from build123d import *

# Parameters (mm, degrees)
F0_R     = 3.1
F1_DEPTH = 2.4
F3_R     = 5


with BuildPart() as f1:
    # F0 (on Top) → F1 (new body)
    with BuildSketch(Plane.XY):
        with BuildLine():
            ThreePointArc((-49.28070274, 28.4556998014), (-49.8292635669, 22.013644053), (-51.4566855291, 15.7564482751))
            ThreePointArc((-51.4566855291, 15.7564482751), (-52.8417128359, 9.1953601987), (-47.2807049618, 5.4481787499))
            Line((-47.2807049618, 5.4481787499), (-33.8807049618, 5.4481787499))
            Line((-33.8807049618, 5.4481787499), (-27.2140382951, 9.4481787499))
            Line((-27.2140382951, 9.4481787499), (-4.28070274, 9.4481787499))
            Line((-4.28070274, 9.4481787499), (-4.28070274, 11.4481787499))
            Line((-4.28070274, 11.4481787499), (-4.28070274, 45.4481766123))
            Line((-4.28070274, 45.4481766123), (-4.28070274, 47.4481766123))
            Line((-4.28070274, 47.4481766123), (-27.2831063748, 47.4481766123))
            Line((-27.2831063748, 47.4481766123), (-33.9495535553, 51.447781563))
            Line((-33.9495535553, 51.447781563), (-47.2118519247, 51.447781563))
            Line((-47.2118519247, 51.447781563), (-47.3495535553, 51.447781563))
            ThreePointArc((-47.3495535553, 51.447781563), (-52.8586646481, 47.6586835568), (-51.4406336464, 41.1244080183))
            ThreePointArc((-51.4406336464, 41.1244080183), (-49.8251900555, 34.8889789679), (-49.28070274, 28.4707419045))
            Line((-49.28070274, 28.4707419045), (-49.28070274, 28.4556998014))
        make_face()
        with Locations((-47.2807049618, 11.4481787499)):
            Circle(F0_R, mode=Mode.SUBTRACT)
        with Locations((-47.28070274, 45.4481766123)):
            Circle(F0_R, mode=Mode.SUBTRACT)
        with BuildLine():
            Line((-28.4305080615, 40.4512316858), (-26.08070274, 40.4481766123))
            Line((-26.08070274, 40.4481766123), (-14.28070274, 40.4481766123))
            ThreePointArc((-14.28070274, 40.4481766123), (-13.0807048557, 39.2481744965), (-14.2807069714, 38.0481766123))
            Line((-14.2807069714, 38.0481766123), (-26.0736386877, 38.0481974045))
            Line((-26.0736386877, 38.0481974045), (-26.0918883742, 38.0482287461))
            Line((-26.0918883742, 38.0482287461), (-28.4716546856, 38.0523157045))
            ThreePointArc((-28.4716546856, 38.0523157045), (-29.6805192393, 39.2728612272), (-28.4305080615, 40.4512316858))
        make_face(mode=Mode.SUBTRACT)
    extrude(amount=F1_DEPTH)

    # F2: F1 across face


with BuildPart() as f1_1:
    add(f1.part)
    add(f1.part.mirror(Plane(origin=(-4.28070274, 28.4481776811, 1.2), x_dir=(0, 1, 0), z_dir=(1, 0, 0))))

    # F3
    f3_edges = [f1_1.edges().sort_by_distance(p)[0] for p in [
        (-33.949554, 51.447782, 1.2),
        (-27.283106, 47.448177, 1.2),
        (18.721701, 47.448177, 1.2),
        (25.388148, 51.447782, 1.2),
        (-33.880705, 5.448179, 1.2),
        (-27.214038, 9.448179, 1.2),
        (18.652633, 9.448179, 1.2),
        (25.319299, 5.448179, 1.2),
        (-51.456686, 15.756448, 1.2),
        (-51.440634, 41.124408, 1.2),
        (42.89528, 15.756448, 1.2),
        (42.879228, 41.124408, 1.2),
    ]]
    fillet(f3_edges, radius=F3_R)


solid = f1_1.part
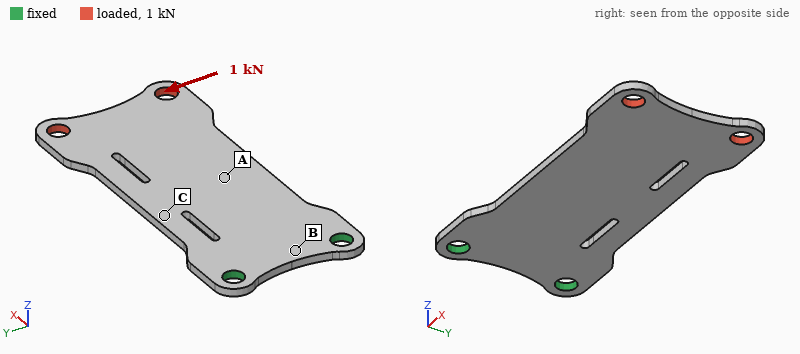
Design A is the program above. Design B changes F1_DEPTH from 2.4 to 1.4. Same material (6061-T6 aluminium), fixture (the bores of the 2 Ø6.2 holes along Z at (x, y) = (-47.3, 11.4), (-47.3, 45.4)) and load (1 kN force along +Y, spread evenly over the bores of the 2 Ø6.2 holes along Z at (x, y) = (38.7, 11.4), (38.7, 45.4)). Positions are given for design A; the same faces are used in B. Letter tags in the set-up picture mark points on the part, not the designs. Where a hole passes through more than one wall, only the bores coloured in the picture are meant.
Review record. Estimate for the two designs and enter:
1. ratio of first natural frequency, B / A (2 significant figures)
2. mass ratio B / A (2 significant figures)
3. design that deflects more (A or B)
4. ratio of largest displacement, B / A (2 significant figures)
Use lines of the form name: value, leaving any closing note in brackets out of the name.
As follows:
ratio of first natural frequency, B / A: 0.59
mass ratio B / A: 0.58
design that deflects more: B
ratio of largest displacement, B / A: 1.7
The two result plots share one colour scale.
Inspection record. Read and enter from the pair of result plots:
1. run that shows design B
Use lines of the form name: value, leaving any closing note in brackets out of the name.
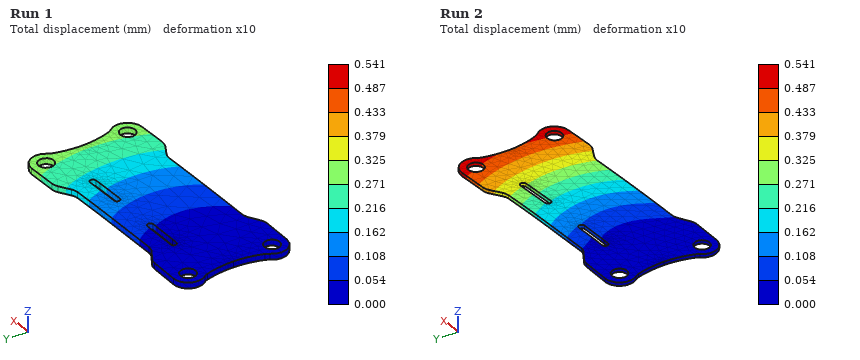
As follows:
run that shows design B: Run 2
